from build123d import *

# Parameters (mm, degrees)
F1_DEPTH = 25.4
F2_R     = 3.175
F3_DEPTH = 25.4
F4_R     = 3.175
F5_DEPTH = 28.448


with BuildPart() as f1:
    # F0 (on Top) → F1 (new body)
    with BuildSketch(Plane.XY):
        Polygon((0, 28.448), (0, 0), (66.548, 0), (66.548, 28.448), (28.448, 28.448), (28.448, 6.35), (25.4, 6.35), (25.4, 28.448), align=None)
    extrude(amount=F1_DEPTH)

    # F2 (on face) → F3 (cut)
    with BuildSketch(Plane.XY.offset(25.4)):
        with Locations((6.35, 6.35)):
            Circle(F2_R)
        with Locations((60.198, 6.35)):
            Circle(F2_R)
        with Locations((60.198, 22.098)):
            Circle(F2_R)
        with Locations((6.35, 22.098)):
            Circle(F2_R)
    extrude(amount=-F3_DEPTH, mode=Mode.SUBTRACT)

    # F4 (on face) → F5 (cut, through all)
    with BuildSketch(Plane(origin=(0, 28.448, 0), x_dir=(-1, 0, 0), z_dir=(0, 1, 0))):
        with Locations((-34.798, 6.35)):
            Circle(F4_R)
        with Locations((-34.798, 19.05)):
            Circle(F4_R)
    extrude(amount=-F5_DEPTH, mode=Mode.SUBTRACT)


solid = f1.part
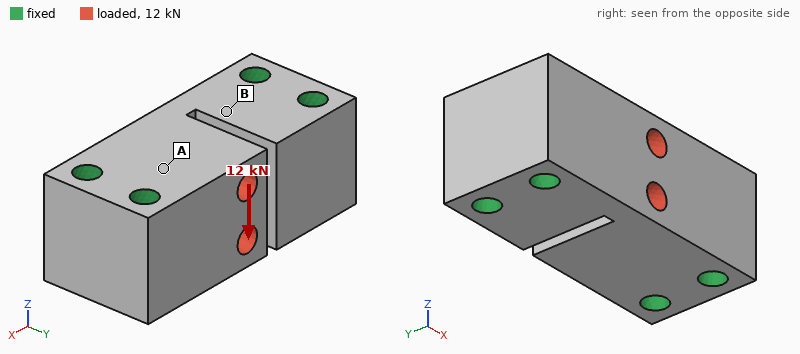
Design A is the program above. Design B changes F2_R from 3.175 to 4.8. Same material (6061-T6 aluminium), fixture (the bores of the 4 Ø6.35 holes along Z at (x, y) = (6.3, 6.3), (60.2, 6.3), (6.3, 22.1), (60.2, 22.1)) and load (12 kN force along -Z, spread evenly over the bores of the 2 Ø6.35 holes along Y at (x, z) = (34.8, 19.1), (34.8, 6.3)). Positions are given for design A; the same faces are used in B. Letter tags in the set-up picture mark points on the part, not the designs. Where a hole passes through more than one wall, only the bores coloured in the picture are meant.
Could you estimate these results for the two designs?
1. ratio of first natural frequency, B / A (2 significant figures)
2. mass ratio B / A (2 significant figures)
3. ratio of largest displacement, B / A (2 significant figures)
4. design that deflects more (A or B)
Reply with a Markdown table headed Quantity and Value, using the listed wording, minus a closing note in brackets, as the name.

| Quantity | Value |
|---|---|
| ratio of first natural frequency, B / A | 1.1 |
| mass ratio B / A | 0.90 |
| ratio of largest displacement, B / A | 0.88 |
| design that deflects more | A |
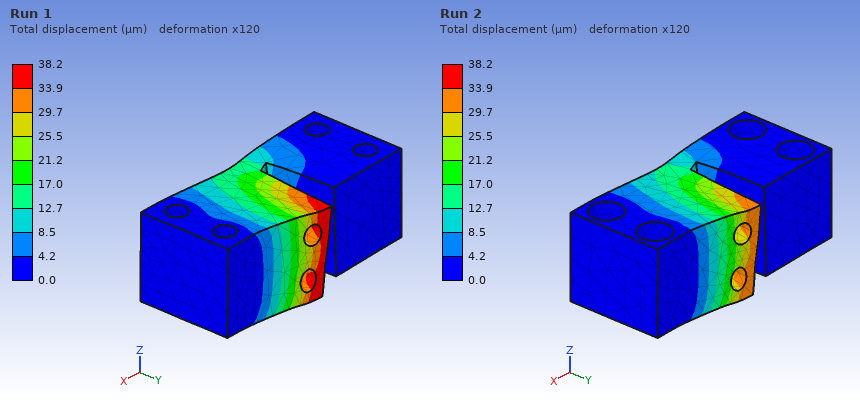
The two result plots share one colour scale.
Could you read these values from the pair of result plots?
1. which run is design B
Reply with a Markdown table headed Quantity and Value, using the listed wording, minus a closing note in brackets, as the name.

| Quantity | Value |
|---|---|
| which run is design B | Run 2 |
